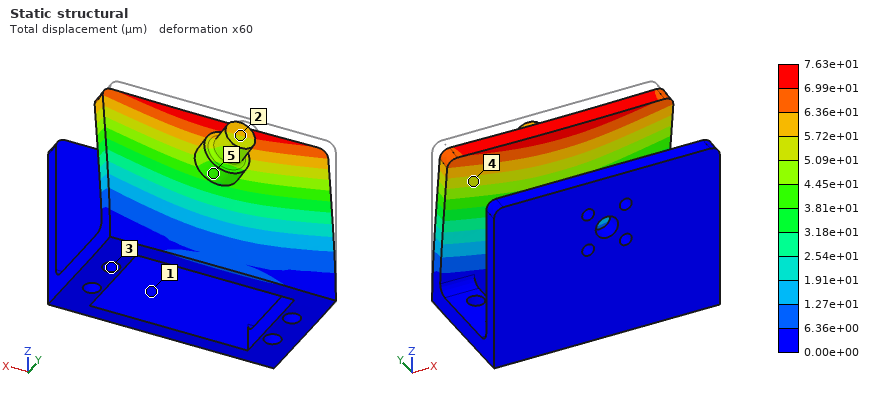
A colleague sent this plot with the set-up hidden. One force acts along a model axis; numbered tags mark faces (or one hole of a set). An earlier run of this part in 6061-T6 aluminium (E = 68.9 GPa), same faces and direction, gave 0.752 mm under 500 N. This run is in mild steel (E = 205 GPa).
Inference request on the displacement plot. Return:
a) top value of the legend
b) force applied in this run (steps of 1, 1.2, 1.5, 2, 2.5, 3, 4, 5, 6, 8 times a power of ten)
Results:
7.63e+01 µm
150 N
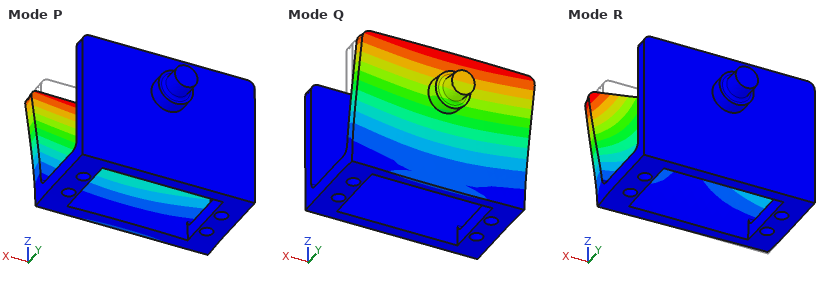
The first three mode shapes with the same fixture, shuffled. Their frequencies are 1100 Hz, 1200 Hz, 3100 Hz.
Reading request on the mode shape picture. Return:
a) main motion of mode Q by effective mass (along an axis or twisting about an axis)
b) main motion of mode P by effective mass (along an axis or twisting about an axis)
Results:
along Y
along Y
